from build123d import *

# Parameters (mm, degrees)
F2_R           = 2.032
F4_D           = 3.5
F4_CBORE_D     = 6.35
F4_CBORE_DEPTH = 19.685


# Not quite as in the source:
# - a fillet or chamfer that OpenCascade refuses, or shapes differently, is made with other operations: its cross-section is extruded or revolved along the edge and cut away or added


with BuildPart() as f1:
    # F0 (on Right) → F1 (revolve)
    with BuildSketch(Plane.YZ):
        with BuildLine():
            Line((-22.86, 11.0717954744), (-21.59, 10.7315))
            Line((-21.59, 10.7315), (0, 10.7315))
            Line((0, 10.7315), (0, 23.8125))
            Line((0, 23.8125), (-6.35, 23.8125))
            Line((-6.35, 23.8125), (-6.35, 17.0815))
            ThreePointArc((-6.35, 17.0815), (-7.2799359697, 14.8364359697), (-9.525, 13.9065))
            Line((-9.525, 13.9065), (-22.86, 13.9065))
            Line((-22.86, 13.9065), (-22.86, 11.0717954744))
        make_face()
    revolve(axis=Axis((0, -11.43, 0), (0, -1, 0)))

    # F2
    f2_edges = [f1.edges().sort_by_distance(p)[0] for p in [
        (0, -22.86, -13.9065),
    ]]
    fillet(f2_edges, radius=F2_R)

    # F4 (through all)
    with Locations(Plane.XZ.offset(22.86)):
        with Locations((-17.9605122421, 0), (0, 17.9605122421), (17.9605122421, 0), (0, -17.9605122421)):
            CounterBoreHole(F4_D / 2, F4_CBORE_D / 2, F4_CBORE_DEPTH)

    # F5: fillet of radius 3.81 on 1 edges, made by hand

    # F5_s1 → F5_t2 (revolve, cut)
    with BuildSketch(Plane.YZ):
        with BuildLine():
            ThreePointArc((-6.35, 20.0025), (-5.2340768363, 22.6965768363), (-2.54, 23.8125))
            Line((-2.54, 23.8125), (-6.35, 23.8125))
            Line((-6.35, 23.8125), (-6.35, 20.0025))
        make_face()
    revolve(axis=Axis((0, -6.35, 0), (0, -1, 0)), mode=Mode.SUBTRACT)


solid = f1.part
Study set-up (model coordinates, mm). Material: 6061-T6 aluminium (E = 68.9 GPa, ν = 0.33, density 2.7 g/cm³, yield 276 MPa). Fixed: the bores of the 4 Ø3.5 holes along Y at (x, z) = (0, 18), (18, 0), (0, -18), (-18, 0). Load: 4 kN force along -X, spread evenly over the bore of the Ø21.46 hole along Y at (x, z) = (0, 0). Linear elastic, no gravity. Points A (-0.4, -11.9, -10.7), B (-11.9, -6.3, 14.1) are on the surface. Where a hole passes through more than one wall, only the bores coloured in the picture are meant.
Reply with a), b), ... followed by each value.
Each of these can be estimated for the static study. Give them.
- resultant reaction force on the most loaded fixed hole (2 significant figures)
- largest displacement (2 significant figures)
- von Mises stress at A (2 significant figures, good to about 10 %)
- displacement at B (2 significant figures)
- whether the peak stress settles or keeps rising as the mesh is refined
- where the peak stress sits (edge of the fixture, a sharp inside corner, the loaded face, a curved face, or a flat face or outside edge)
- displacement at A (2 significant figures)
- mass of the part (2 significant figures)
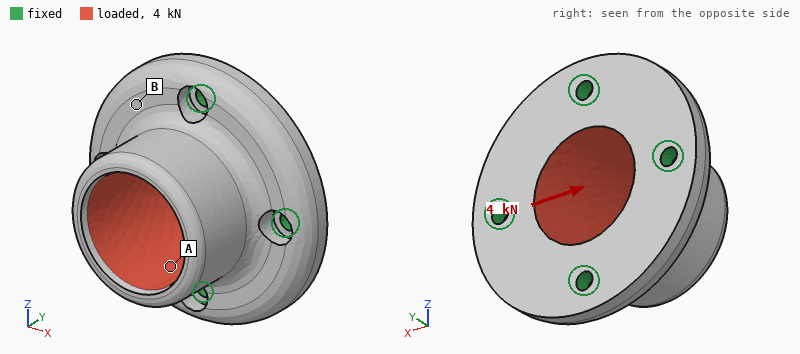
a) 1.5 kN
b) 17 µm
c) 24 MPa
d) 6.1 µm
e) keeps rising
f) edge of the fixture
g) 9.4 µm
h) 33 g
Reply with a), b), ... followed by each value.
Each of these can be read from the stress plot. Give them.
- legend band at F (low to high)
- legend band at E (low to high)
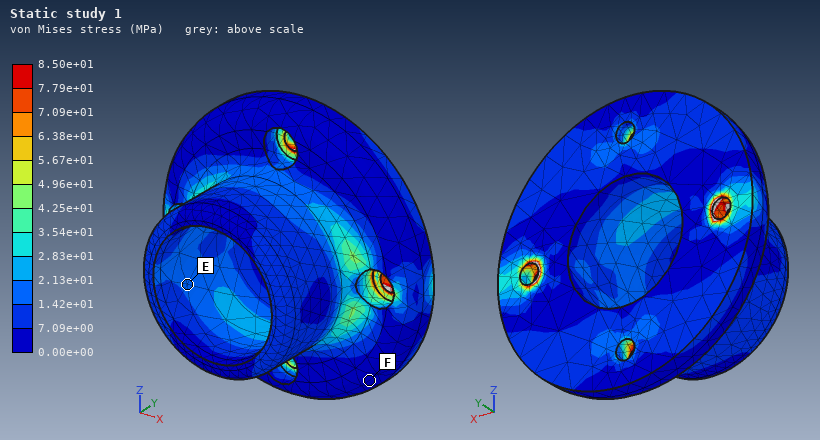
a) 0.00e+00 to 7.09e+00 MPa
b) 1.42e+01 to 2.13e+01 MPa
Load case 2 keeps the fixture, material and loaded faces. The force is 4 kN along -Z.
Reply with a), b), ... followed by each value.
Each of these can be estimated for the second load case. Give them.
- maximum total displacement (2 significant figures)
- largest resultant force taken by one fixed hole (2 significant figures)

a) 17 µm
b) 1.5 kN
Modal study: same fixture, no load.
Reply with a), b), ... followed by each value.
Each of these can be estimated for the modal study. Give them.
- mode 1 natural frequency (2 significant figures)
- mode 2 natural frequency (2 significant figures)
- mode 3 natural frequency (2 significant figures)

a) 17 kHz
b) 19 kHz
c) 19 kHz
